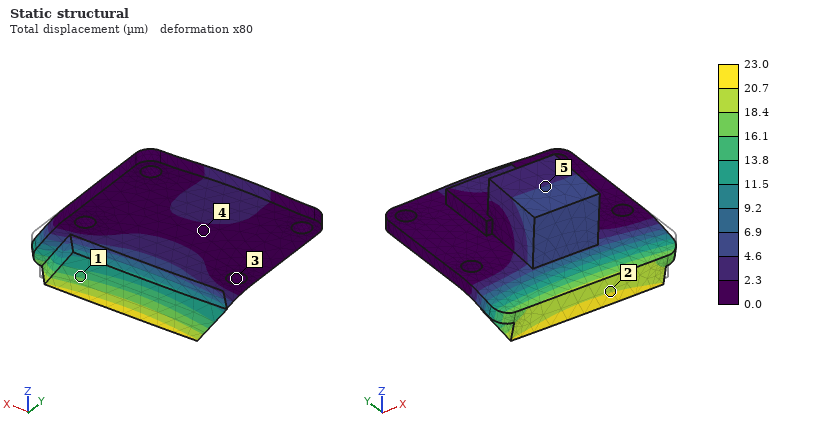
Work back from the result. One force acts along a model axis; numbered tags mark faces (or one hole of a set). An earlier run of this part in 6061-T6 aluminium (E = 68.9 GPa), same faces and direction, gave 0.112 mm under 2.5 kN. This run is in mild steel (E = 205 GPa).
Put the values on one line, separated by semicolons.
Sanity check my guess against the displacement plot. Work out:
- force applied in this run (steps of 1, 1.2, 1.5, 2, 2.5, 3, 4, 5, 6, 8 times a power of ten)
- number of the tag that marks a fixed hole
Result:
1.5 kN; 3
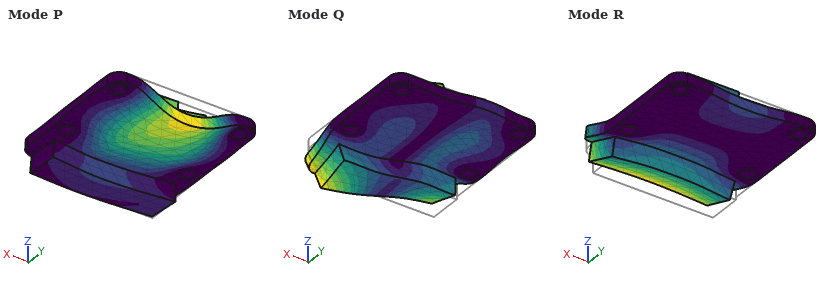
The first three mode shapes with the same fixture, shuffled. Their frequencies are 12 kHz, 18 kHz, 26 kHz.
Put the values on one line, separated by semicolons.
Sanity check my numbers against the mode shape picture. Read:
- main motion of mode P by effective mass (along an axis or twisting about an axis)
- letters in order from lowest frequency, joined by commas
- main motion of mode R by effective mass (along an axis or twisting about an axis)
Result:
along Z; R, P, Q; along Z
